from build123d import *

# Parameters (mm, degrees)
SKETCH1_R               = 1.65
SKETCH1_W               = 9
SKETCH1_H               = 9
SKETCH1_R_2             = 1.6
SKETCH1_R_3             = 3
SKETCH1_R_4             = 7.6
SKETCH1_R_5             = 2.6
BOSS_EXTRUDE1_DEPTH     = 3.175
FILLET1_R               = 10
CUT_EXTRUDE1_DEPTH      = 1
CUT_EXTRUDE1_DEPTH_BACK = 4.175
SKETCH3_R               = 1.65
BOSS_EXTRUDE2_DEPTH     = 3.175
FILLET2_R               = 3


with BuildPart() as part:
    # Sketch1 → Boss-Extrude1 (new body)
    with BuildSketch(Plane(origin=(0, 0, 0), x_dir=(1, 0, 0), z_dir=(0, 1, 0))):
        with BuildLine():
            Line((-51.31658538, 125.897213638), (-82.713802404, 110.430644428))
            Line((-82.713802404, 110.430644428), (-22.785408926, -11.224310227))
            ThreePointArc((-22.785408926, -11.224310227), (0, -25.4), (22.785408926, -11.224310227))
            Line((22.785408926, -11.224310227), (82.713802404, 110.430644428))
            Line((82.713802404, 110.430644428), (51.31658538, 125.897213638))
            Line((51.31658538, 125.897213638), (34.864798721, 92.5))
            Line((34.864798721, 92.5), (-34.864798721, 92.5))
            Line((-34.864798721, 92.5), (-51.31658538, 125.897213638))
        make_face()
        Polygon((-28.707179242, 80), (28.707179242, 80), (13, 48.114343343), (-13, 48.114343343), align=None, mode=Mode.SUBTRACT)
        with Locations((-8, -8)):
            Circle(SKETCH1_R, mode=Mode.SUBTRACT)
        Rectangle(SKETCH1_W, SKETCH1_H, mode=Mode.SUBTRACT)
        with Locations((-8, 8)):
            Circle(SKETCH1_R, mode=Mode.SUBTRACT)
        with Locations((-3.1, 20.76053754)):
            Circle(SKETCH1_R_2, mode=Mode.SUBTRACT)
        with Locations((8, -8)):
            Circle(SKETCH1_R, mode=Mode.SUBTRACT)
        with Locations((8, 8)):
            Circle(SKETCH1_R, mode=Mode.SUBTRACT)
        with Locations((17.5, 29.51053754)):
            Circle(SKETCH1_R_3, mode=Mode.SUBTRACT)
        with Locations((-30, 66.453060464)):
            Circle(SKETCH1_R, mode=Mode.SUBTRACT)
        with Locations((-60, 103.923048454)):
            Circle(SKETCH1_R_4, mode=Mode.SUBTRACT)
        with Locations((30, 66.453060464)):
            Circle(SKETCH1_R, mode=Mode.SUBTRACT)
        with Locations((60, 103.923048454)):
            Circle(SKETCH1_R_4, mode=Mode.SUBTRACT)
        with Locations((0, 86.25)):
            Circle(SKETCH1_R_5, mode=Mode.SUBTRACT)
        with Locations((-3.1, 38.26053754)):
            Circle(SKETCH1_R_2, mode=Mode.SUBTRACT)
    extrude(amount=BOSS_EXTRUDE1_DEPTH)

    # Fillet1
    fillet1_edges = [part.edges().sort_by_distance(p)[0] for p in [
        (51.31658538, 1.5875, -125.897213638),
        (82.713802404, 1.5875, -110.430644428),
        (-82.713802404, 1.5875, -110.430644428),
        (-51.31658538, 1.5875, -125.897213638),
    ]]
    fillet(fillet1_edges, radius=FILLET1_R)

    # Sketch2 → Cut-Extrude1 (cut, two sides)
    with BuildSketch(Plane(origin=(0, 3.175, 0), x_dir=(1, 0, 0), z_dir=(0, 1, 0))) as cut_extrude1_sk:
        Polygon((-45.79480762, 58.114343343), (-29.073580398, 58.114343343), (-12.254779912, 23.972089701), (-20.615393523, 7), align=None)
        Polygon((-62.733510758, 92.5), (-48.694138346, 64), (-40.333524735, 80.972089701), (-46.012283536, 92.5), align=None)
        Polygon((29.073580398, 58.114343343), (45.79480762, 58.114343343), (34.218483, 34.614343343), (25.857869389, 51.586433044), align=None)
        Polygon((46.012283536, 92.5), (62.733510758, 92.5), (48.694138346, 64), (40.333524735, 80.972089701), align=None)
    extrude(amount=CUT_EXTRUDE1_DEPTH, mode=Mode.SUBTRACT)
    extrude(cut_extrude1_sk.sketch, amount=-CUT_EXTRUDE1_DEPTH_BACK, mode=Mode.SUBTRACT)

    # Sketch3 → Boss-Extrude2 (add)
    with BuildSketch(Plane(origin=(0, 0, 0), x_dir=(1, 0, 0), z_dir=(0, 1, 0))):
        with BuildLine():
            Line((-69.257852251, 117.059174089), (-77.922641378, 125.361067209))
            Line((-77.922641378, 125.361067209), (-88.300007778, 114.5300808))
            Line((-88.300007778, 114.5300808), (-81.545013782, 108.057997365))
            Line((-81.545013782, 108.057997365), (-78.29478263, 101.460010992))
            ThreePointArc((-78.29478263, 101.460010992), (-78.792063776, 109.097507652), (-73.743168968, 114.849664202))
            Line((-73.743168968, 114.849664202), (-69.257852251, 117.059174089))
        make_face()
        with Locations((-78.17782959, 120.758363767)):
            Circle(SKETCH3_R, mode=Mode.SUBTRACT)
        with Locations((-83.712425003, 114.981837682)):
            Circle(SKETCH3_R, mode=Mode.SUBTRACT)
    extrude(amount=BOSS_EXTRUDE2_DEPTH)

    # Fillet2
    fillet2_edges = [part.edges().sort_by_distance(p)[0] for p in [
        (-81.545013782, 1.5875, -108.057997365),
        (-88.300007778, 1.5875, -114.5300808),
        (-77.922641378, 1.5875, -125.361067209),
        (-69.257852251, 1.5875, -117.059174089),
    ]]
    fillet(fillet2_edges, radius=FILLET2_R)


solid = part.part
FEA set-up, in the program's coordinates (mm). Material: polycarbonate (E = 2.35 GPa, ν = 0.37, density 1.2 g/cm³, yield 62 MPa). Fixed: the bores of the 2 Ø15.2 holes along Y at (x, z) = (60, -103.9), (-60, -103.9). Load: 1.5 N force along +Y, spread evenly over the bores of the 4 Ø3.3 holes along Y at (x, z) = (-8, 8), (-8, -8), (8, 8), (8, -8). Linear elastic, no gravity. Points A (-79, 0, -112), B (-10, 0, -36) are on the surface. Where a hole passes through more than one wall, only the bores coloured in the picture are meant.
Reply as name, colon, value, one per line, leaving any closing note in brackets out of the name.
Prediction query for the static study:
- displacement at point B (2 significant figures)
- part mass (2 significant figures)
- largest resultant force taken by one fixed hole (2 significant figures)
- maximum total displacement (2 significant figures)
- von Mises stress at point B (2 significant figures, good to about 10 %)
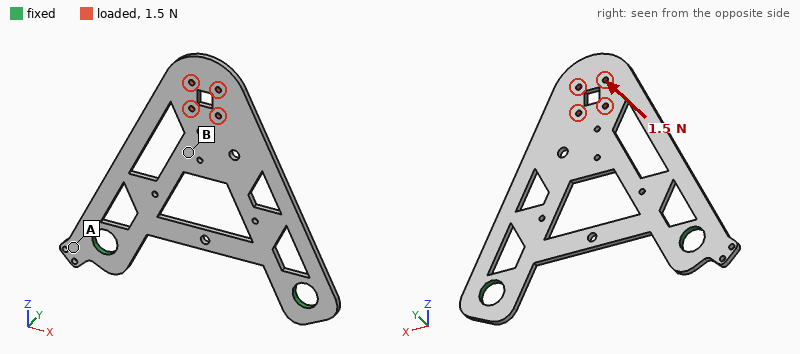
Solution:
displacement at point B: 0.99 mm
part mass: 34 g
largest resultant force taken by one fixed hole: 0.77 N
maximum total displacement: 2.6 mm
von Mises stress at point B: 0.53 MPa
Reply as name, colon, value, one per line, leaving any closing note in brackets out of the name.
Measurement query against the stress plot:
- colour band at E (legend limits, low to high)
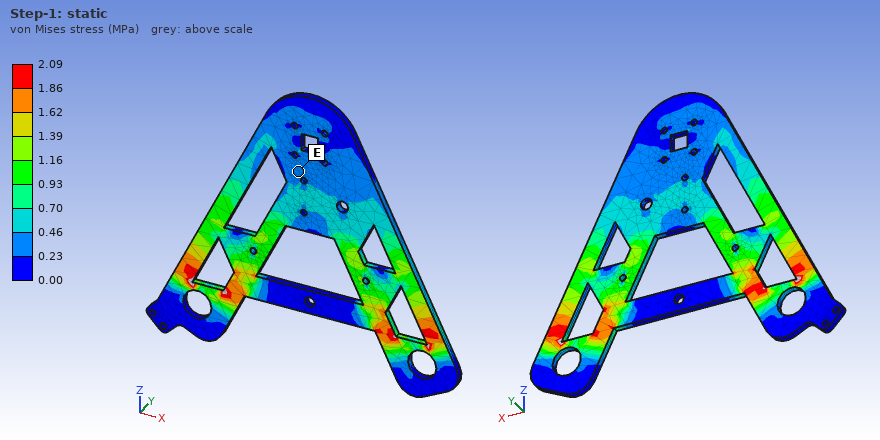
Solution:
colour band at E: 0.23 to 0.46 MPa
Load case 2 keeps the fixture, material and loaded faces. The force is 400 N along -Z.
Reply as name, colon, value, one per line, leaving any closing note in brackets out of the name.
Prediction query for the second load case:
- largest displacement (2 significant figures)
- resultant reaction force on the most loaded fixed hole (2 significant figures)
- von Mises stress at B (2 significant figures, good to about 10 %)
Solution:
largest displacement: 0.19 mm
resultant reaction force on the most loaded fixed hole: 230 N
von Mises stress at B: 2.5 MPa
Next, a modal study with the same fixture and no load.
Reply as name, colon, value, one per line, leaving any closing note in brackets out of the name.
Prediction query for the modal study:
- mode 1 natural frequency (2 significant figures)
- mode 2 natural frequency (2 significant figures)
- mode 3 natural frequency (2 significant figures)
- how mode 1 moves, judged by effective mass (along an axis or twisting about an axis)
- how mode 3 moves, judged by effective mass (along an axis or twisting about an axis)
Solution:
mode 1 natural frequency: 43 Hz
mode 2 natural frequency: 200 Hz
mode 3 natural frequency: 240 Hz
how mode 1 moves, judged by effective mass: along Y
how mode 3 moves, judged by effective mass: along Y
